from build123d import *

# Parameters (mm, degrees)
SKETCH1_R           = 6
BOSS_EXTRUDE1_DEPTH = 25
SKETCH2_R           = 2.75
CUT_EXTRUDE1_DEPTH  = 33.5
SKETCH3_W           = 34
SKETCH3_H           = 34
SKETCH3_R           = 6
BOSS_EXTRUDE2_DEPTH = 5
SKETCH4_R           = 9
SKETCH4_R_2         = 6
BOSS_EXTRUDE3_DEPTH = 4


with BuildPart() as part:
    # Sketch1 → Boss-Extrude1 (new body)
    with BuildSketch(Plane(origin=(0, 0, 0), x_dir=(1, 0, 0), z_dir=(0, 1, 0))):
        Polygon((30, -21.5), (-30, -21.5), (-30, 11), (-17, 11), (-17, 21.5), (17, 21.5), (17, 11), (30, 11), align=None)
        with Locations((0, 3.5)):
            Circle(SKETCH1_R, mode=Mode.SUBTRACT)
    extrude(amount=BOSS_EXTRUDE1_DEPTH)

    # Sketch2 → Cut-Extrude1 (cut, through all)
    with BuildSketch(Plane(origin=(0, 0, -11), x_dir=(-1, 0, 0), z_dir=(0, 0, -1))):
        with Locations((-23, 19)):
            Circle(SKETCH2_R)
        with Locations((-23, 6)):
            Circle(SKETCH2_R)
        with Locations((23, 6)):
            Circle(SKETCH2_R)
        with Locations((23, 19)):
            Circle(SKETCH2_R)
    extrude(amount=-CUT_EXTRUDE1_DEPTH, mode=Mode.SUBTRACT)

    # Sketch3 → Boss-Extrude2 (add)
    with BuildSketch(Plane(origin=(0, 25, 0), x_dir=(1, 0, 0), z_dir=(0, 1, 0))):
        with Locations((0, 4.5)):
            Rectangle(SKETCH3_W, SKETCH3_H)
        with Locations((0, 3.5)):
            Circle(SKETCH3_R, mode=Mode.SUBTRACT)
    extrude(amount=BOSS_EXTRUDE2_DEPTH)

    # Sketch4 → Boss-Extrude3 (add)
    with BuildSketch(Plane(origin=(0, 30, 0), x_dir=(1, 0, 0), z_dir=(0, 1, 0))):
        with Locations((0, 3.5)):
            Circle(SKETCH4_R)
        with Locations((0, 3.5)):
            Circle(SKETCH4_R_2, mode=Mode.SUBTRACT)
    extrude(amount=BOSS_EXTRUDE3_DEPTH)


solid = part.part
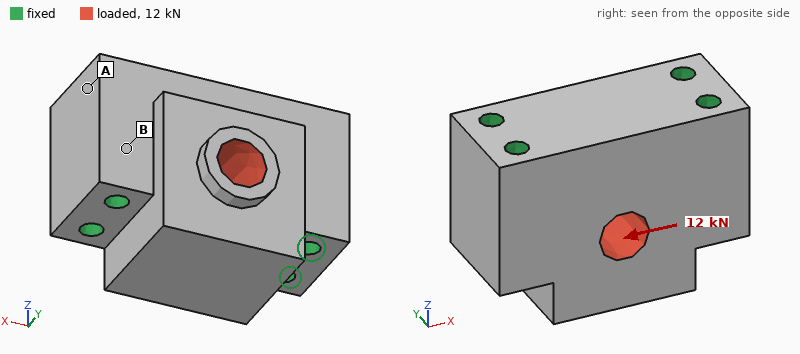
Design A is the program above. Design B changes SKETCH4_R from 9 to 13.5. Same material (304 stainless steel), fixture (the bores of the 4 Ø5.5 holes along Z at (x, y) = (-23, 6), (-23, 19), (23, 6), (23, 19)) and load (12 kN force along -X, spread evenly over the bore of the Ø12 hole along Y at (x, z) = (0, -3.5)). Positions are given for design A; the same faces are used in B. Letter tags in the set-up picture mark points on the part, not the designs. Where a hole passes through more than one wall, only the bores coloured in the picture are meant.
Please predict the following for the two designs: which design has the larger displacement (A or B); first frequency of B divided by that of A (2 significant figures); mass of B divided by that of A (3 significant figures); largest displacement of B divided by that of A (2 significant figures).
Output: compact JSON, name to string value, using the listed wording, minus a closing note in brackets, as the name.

{"which design has the larger displacement": "A", "first frequency of B divided by that of A": "0.98", "mass of B divided by that of A": "1.02", "largest displacement of B divided by that of A": "0.71"}
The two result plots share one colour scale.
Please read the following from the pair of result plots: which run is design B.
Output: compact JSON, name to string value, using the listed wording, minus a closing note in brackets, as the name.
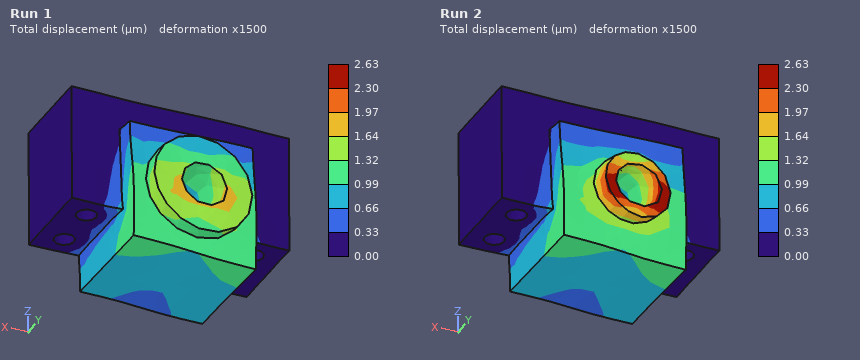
{"which run is design B": "Run 1"}
